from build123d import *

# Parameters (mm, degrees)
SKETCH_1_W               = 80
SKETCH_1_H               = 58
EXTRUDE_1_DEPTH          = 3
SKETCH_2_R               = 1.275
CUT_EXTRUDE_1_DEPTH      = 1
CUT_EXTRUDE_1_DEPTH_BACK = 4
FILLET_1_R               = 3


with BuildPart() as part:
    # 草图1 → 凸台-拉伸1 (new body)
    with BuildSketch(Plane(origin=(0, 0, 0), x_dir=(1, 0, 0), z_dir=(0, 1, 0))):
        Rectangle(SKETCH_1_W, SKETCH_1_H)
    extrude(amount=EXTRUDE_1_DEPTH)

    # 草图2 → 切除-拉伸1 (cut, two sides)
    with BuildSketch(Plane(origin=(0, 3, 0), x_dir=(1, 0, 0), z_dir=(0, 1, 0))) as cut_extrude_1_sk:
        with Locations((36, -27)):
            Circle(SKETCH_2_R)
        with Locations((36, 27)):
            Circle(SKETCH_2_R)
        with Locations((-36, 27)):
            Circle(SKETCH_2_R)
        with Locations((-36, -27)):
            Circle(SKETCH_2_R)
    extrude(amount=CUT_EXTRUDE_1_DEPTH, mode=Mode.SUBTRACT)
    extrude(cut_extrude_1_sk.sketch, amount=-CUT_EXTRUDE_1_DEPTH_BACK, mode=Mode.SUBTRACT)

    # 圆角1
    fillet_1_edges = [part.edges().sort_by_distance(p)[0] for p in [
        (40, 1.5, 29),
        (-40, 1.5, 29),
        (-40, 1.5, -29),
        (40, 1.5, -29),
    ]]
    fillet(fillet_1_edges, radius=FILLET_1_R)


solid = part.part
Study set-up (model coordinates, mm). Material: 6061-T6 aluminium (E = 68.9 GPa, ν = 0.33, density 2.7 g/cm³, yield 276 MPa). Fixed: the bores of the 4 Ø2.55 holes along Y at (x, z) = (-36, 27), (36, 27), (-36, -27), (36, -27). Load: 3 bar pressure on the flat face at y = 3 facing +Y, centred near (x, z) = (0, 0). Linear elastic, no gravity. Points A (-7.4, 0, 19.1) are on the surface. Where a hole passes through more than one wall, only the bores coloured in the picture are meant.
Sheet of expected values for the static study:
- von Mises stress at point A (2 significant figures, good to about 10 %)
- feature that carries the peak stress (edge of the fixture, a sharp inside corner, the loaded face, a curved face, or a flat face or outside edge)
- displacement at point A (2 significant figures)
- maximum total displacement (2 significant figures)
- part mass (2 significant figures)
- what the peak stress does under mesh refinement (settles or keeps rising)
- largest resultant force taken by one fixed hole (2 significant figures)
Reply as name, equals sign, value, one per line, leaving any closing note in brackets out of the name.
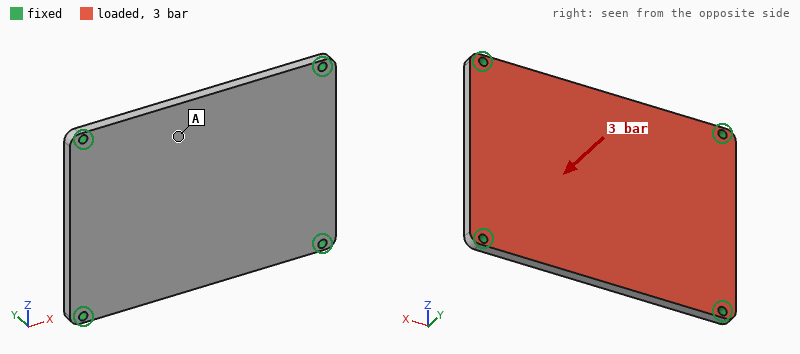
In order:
von Mises stress at point A = 53 MPa
feature that carries the peak stress = edge of the fixture
displacement at point A = 0.24 mm
maximum total displacement = 0.28 mm
part mass = 37 g
what the peak stress does under mesh refinement = keeps rising
largest resultant force taken by one fixed hole = 350 N
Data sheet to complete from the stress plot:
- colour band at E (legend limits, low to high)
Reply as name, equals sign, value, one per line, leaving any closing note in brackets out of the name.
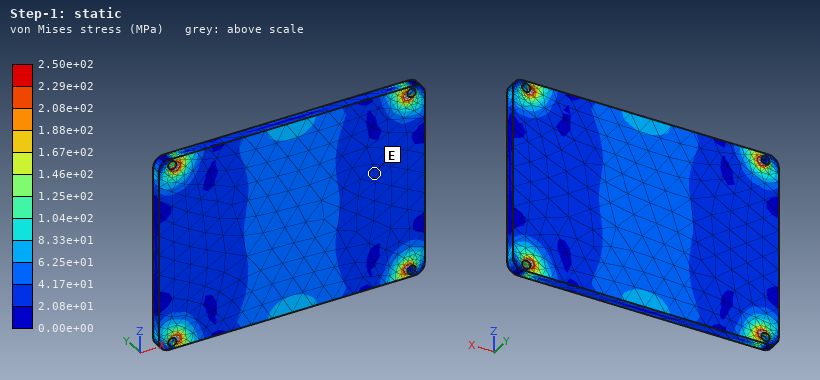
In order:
colour band at E = 2.08e+01 to 4.17e+01 MPa
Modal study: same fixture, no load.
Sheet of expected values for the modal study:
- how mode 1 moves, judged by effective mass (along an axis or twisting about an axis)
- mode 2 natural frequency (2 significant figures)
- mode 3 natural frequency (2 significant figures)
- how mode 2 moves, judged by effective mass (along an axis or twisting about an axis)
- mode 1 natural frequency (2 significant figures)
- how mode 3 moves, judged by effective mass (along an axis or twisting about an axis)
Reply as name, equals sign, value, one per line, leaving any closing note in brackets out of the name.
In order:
how mode 1 moves, judged by effective mass = along Y
mode 2 natural frequency = 3700 Hz
mode 3 natural frequency = 4800 Hz
how mode 2 moves, judged by effective mass = twisting about X
mode 1 natural frequency = 2100 Hz
how mode 3 moves, judged by effective mass = twisting about Z
